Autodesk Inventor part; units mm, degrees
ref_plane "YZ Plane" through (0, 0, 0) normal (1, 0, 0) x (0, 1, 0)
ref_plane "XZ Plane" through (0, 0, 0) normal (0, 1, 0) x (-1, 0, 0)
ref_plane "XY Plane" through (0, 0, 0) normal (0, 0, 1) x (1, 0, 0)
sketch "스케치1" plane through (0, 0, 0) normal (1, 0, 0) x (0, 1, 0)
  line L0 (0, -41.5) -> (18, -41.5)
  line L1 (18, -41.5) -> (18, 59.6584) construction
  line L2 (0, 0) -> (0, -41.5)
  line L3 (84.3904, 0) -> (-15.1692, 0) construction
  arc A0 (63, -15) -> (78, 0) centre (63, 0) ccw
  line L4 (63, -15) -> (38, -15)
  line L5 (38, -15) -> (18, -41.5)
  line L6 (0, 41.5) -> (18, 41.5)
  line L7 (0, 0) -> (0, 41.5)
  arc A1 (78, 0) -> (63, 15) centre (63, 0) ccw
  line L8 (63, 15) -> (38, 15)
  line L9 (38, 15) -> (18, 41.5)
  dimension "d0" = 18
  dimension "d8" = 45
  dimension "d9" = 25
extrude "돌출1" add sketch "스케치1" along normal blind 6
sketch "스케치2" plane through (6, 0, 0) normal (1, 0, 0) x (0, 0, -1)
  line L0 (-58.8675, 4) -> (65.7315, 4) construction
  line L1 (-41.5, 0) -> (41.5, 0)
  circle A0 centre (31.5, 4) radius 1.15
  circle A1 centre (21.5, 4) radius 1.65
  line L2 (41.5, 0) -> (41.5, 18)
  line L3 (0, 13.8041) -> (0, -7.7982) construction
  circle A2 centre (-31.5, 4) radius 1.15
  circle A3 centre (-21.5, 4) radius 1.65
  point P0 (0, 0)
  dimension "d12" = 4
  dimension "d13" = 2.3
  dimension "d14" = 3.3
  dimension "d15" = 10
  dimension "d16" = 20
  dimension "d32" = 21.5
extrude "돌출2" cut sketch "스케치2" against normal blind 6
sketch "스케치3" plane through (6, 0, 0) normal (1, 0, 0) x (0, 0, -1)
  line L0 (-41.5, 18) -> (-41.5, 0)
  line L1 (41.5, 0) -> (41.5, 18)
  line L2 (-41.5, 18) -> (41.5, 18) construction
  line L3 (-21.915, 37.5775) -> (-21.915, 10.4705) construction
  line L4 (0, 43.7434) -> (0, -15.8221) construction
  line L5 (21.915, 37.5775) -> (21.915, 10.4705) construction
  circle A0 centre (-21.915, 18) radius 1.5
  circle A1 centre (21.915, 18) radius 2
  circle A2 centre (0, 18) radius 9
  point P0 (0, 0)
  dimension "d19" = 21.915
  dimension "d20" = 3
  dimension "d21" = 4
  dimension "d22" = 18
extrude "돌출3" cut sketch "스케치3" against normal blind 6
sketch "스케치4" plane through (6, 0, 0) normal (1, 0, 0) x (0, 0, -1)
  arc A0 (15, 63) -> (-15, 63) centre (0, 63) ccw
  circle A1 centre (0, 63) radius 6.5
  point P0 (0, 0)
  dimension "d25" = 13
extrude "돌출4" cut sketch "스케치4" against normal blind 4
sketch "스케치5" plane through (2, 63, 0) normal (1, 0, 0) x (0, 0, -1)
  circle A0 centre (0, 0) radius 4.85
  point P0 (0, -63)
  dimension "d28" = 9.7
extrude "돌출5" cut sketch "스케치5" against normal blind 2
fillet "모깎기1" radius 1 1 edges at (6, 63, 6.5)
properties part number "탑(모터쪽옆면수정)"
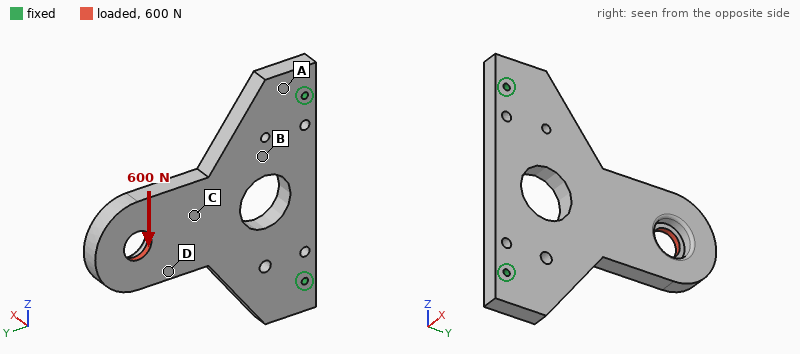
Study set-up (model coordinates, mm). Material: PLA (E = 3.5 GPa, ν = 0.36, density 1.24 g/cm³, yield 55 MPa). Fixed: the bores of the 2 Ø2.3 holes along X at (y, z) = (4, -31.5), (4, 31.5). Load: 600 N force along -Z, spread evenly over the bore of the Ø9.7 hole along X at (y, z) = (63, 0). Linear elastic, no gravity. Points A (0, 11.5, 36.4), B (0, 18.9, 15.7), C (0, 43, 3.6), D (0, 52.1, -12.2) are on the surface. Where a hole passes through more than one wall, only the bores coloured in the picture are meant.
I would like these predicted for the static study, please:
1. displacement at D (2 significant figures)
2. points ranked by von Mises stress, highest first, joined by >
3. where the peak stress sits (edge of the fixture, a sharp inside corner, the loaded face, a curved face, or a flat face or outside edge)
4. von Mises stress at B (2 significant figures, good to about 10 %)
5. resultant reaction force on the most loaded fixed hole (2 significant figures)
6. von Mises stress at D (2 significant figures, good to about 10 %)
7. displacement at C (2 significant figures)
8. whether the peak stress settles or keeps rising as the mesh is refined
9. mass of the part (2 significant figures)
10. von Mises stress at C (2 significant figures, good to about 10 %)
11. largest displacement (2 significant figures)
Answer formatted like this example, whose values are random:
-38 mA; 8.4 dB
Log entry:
0.34 mm; C > D > B > A; edge of the fixture; 5.6 MPa; 630 N; 10 MPa; 0.17 mm; keeps rising; 25 g; 13 MPa; 0.62 mm
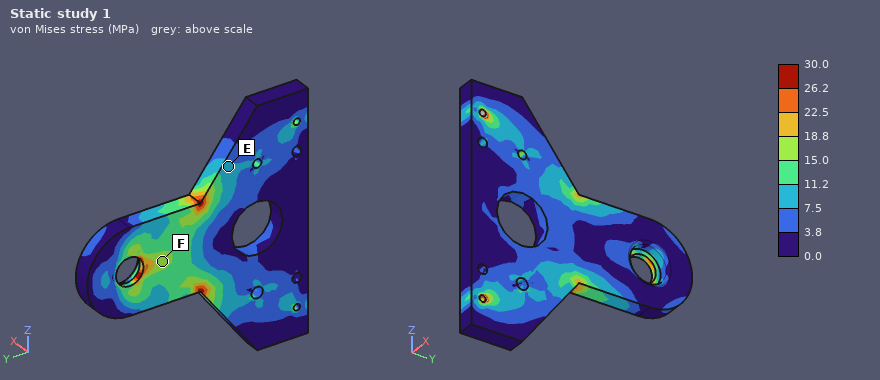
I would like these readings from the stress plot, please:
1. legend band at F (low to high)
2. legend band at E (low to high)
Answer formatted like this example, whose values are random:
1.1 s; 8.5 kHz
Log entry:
15.0 to 18.8 MPa; 7.5 to 11.2 MPa
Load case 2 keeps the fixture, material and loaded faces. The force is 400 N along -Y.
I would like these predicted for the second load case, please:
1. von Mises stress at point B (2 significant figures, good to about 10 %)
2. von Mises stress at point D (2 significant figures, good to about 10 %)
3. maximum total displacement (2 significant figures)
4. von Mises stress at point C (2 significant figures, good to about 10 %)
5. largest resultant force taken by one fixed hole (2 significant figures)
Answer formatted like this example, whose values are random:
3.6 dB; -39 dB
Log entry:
4.9 MPa; 6.4 MPa; 1.1 mm; 5.8 MPa; 230 N
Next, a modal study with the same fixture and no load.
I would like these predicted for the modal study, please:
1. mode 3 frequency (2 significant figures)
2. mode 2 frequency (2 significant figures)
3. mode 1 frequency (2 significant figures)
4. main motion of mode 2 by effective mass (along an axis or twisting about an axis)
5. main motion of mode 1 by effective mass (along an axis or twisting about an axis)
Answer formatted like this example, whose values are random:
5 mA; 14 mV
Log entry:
1700 Hz; 1500 Hz; 330 Hz; along X; along X
